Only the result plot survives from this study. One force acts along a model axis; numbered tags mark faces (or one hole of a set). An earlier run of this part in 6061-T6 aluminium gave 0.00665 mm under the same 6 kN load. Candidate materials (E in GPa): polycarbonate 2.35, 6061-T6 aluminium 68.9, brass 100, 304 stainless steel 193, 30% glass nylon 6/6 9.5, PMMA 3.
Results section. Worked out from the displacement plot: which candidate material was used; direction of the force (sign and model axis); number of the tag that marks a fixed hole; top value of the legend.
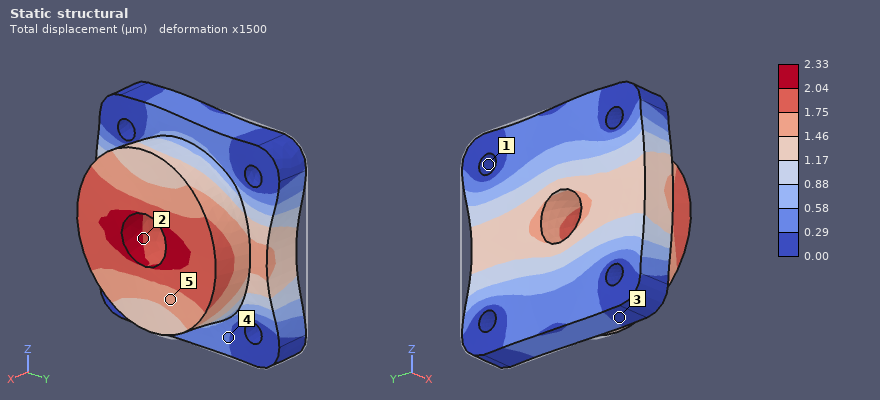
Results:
304 stainless steel
-Y
1
2.33 µm
